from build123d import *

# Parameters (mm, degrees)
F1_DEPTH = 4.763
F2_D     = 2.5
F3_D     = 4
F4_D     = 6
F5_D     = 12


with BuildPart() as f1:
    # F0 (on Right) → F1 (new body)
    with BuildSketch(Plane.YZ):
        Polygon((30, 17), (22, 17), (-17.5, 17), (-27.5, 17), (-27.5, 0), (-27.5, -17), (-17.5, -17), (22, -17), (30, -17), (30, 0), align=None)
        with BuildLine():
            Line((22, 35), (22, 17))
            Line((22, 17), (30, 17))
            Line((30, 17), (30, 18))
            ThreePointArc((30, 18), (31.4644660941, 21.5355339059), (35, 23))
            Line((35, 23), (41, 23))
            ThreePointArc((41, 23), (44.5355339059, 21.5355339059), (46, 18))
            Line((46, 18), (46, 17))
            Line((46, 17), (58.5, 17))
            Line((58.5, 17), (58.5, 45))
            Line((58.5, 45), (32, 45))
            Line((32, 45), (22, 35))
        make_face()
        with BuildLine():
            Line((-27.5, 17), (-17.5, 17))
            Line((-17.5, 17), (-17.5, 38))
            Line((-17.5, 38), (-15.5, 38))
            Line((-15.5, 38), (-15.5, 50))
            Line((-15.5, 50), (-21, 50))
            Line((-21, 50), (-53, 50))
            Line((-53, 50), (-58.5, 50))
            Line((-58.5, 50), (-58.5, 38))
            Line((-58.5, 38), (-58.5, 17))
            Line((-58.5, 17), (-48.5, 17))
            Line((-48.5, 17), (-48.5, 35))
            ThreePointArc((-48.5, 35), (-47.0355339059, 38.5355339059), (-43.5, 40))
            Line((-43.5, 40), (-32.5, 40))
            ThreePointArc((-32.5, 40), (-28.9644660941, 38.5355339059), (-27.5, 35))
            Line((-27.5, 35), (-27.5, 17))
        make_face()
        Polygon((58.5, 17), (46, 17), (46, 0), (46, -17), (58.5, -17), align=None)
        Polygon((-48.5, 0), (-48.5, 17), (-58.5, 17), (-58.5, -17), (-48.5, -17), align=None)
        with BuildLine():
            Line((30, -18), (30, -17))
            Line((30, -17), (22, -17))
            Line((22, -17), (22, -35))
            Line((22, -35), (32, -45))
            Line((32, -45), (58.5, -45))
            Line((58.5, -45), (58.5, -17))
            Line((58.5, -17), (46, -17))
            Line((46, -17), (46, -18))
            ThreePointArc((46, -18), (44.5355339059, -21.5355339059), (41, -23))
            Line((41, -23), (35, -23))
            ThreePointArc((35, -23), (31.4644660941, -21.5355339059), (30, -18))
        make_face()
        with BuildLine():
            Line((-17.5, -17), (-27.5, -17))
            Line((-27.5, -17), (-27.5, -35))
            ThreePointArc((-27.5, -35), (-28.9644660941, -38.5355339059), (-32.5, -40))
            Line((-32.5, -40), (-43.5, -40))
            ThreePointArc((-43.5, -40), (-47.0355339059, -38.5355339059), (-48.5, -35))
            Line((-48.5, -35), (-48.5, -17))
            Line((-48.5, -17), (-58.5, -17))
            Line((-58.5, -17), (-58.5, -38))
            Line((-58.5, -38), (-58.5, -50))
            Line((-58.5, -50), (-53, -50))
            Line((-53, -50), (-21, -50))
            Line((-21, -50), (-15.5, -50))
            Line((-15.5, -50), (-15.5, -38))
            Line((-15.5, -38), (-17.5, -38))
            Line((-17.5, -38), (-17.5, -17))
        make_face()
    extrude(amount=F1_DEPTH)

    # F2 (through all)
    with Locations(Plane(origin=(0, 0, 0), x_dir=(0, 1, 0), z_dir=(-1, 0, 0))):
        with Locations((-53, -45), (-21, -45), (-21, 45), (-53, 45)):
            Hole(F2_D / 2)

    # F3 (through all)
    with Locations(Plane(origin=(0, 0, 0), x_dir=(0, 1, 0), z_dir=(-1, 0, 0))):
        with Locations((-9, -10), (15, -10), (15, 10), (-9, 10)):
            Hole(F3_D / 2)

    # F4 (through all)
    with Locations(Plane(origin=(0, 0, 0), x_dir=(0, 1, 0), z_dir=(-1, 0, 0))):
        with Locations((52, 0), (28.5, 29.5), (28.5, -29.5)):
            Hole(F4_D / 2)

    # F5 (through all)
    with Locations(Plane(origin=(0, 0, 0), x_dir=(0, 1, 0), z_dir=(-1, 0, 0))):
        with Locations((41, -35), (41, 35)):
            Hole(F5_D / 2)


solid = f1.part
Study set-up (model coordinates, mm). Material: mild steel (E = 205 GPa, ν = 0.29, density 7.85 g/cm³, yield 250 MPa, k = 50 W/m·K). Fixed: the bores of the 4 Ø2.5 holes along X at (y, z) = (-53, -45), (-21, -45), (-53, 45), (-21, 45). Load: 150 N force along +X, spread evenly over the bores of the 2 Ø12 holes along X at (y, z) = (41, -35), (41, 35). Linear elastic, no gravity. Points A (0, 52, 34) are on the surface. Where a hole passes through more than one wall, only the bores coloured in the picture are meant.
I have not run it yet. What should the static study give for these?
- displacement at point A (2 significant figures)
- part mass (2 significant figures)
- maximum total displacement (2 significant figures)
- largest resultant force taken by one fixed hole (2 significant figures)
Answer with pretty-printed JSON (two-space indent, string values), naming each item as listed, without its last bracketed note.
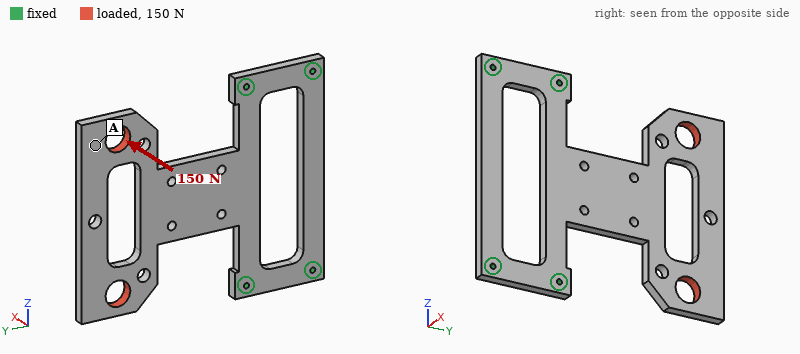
{
  "displacement at point A": "0.80 mm",
  "part mass": "220 g",
  "maximum total displacement": "0.90 mm",
  "largest resultant force taken by one fixed hole": "150 N"
}
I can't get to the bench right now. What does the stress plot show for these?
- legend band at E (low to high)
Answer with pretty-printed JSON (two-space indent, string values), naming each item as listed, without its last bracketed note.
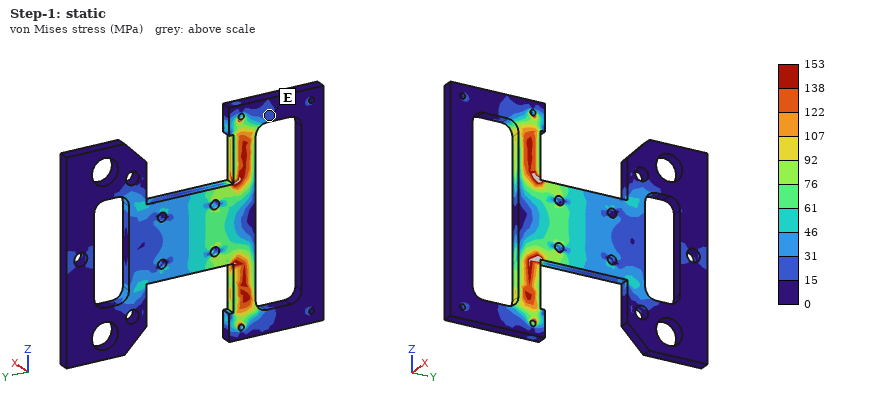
{
  "legend band at E": "15 to 31 MPa"
}
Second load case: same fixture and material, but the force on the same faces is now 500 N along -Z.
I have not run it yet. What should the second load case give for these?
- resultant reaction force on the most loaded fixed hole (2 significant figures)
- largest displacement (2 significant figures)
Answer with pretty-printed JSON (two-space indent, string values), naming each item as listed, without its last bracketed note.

{
  "resultant reaction force on the most loaded fixed hole": "370 N",
  "largest displacement": "0.11 mm"
}
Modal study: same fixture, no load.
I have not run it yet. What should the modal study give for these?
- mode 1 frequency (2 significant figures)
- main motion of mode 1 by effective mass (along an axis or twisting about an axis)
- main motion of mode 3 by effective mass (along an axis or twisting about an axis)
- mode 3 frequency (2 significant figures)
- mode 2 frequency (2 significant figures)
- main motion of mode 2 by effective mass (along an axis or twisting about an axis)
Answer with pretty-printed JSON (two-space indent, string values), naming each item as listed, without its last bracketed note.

{
  "mode 1 frequency": "250 Hz",
  "main motion of mode 1 by effective mass": "along X",
  "main motion of mode 3 by effective mass": "along Z",
  "mode 3 frequency": "1300 Hz",
  "mode 2 frequency": "720 Hz",
  "main motion of mode 2 by effective mass": "twisting about Y"
}
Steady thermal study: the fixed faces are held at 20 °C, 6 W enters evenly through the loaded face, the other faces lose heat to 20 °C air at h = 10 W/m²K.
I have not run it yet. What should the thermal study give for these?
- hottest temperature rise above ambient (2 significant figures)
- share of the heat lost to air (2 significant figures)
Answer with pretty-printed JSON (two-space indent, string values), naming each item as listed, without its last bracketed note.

{
  "hottest temperature rise above ambient": "53 K",
  "share of the heat lost to air": "63 %"
}
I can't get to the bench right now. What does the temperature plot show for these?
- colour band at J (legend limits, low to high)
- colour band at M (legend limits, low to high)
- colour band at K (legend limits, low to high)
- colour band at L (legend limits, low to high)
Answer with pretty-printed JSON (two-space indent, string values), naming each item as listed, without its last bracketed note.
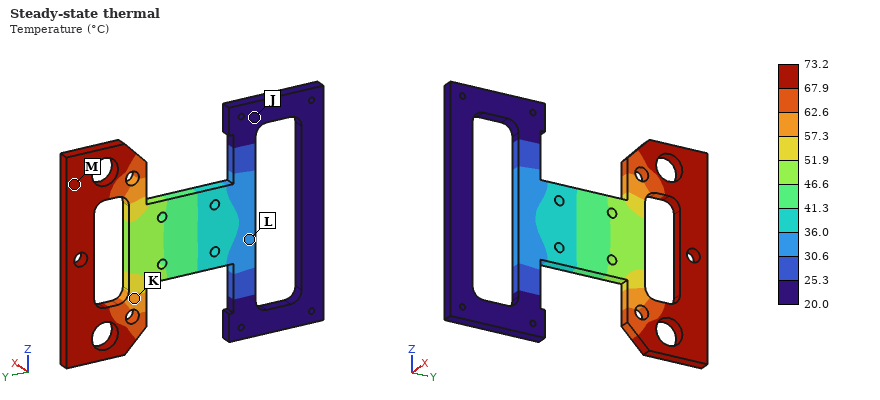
{
  "colour band at J": "20.0 to 25.3 °C",
  "colour band at M": "67.9 to 73.2 °C",
  "colour band at K": "57.3 to 62.6 °C",
  "colour band at L": "30.6 to 36.0 °C"
}
